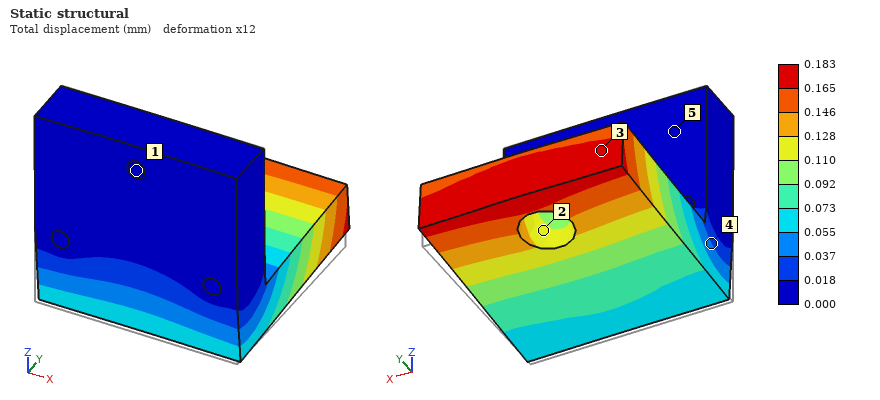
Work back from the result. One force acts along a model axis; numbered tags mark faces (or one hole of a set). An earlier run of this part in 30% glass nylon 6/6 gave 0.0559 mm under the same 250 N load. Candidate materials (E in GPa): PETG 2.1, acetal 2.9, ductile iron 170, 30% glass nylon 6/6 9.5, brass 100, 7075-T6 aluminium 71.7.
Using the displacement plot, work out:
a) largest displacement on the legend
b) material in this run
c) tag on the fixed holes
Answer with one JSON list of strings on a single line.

["0.183 mm", "acetal", "1"]
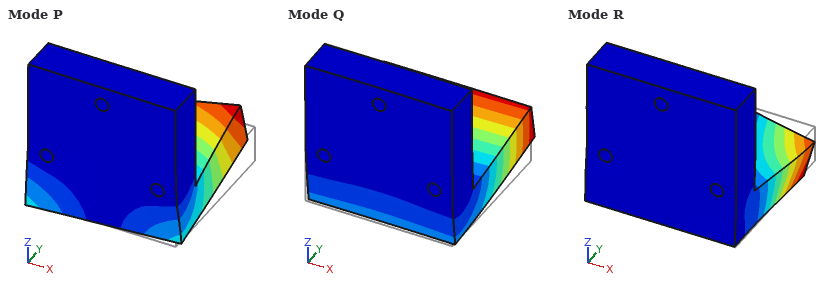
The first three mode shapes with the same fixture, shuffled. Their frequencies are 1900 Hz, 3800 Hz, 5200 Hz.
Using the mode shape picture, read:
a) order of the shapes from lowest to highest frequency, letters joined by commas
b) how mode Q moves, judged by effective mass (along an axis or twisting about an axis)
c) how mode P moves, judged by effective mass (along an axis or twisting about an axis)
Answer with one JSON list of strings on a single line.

["Q, P, R", "along Z", "along X"]
